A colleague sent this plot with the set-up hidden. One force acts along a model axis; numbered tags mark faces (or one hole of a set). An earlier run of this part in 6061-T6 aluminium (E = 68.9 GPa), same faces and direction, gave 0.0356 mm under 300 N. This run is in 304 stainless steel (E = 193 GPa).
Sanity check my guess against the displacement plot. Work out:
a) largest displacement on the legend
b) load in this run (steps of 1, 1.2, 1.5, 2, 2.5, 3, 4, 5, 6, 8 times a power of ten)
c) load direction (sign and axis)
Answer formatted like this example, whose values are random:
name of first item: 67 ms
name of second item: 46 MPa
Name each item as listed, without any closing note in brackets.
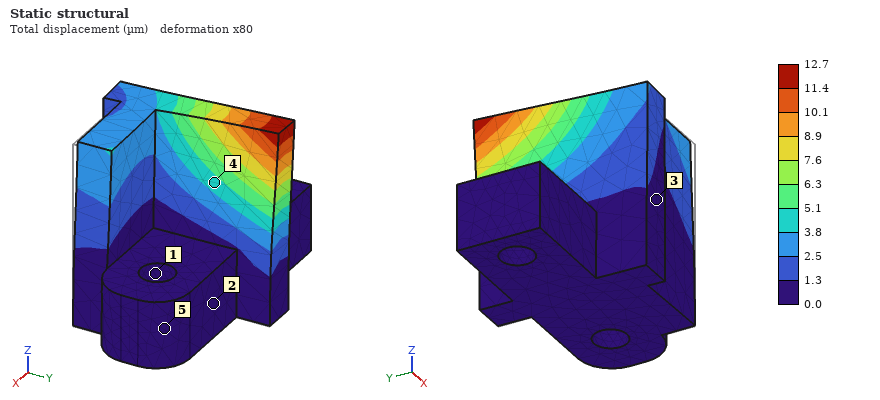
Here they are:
largest displacement on the legend: 12.7 µm
load in this run: 300 N
load direction: -X
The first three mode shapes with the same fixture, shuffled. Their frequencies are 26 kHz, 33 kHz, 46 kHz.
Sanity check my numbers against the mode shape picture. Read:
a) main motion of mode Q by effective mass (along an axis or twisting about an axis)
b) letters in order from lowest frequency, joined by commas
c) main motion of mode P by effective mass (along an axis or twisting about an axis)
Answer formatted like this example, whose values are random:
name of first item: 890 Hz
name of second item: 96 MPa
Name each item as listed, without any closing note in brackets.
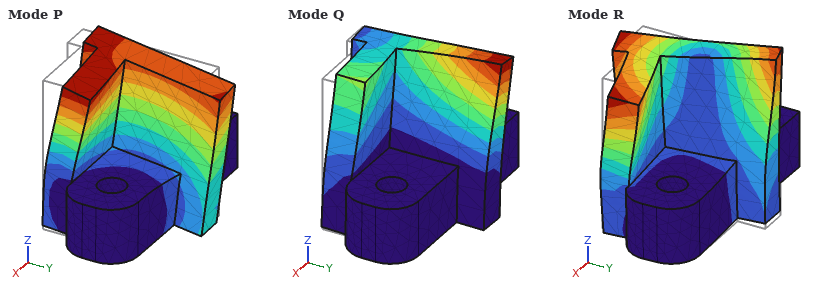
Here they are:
main motion of mode Q by effective mass: along X
letters in order from lowest frequency, joined by commas: P, Q, R
main motion of mode P by effective mass: along Y
